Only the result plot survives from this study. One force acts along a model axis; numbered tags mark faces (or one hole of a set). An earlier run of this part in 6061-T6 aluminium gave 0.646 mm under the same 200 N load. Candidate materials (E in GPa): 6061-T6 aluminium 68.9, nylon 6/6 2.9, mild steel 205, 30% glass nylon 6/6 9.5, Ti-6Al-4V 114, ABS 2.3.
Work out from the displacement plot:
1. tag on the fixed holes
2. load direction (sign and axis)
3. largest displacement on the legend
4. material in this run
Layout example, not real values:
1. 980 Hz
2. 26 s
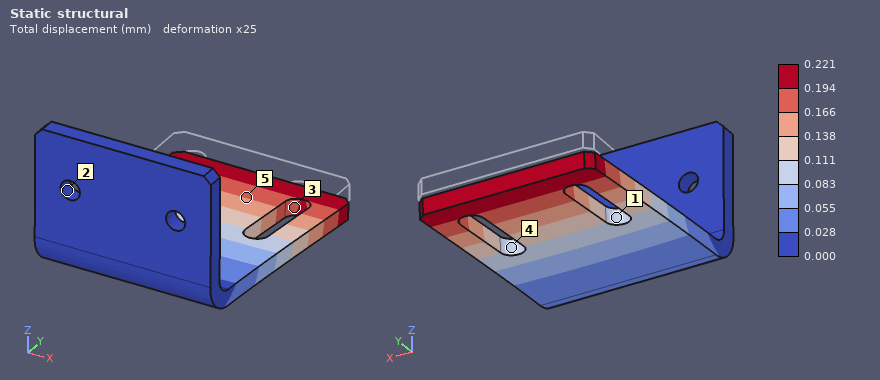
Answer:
1. 2
2. -Z
3. 0.221 mm
4. mild steel
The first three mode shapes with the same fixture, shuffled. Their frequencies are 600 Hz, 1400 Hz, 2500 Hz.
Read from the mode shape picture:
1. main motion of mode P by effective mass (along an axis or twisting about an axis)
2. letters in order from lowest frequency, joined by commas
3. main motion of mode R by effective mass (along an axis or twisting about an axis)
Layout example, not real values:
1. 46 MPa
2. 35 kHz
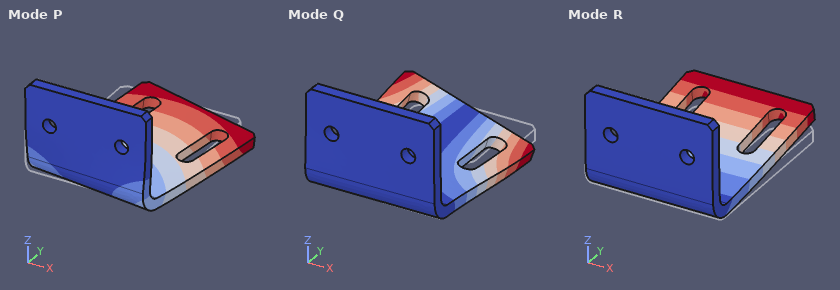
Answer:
1. along X
2. R, P, Q
3. along Z
